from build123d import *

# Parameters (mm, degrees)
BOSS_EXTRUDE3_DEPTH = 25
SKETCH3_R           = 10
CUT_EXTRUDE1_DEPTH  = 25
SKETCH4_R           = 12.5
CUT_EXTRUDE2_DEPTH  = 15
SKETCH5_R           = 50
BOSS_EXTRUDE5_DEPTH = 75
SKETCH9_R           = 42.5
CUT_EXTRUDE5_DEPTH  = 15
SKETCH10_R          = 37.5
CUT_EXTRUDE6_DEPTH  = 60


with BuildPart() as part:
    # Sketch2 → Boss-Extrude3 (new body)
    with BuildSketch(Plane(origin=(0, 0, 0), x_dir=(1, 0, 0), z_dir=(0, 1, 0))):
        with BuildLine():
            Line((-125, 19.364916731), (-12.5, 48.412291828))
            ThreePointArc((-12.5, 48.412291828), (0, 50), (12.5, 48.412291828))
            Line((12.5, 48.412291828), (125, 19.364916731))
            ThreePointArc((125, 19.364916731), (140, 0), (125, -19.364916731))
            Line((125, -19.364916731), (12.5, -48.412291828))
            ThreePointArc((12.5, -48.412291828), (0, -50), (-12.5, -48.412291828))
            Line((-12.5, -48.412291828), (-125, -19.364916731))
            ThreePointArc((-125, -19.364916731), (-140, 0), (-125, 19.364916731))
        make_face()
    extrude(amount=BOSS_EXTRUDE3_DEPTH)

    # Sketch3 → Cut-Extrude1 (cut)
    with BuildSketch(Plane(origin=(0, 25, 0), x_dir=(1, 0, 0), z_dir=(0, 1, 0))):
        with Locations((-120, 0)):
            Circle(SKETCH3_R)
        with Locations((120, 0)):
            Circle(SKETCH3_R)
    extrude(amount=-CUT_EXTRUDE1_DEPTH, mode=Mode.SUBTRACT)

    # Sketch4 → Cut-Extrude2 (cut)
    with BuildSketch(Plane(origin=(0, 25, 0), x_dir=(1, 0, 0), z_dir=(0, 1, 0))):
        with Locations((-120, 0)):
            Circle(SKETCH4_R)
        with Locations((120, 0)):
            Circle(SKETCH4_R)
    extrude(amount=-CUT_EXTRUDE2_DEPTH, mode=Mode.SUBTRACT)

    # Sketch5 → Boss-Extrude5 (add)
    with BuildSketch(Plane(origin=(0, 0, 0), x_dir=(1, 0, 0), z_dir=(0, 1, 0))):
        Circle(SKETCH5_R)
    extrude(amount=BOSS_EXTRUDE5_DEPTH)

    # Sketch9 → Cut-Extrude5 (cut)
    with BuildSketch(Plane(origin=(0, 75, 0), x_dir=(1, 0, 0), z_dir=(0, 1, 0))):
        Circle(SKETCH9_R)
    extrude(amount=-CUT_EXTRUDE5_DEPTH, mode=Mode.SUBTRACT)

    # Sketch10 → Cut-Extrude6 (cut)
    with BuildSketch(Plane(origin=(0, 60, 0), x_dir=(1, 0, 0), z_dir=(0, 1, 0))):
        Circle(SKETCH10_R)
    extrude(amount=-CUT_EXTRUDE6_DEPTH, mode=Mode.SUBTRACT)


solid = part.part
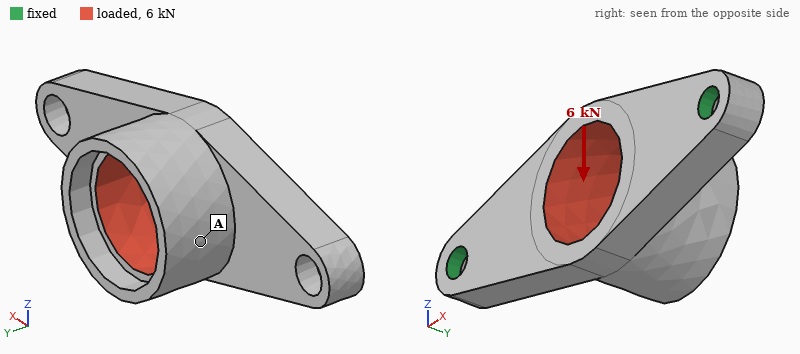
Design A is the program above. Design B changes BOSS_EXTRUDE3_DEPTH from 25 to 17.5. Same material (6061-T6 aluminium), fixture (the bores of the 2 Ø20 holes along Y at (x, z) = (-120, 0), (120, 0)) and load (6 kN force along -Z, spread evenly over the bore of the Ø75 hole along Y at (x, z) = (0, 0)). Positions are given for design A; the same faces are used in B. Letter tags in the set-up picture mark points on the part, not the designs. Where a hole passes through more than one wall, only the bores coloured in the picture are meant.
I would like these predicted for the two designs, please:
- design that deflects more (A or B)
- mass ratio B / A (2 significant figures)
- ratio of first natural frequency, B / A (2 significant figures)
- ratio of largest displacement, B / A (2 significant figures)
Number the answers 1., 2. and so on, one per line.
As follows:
1. B
2. 0.85
3. 0.73
4. 2.0
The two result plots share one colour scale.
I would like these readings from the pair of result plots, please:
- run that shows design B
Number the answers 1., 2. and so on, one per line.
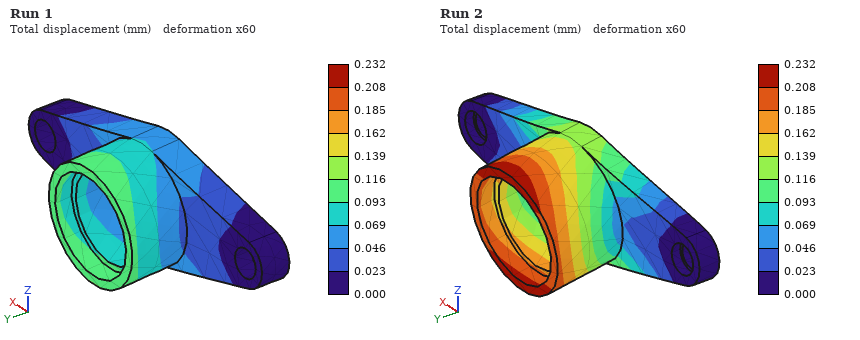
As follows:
1. Run 2
